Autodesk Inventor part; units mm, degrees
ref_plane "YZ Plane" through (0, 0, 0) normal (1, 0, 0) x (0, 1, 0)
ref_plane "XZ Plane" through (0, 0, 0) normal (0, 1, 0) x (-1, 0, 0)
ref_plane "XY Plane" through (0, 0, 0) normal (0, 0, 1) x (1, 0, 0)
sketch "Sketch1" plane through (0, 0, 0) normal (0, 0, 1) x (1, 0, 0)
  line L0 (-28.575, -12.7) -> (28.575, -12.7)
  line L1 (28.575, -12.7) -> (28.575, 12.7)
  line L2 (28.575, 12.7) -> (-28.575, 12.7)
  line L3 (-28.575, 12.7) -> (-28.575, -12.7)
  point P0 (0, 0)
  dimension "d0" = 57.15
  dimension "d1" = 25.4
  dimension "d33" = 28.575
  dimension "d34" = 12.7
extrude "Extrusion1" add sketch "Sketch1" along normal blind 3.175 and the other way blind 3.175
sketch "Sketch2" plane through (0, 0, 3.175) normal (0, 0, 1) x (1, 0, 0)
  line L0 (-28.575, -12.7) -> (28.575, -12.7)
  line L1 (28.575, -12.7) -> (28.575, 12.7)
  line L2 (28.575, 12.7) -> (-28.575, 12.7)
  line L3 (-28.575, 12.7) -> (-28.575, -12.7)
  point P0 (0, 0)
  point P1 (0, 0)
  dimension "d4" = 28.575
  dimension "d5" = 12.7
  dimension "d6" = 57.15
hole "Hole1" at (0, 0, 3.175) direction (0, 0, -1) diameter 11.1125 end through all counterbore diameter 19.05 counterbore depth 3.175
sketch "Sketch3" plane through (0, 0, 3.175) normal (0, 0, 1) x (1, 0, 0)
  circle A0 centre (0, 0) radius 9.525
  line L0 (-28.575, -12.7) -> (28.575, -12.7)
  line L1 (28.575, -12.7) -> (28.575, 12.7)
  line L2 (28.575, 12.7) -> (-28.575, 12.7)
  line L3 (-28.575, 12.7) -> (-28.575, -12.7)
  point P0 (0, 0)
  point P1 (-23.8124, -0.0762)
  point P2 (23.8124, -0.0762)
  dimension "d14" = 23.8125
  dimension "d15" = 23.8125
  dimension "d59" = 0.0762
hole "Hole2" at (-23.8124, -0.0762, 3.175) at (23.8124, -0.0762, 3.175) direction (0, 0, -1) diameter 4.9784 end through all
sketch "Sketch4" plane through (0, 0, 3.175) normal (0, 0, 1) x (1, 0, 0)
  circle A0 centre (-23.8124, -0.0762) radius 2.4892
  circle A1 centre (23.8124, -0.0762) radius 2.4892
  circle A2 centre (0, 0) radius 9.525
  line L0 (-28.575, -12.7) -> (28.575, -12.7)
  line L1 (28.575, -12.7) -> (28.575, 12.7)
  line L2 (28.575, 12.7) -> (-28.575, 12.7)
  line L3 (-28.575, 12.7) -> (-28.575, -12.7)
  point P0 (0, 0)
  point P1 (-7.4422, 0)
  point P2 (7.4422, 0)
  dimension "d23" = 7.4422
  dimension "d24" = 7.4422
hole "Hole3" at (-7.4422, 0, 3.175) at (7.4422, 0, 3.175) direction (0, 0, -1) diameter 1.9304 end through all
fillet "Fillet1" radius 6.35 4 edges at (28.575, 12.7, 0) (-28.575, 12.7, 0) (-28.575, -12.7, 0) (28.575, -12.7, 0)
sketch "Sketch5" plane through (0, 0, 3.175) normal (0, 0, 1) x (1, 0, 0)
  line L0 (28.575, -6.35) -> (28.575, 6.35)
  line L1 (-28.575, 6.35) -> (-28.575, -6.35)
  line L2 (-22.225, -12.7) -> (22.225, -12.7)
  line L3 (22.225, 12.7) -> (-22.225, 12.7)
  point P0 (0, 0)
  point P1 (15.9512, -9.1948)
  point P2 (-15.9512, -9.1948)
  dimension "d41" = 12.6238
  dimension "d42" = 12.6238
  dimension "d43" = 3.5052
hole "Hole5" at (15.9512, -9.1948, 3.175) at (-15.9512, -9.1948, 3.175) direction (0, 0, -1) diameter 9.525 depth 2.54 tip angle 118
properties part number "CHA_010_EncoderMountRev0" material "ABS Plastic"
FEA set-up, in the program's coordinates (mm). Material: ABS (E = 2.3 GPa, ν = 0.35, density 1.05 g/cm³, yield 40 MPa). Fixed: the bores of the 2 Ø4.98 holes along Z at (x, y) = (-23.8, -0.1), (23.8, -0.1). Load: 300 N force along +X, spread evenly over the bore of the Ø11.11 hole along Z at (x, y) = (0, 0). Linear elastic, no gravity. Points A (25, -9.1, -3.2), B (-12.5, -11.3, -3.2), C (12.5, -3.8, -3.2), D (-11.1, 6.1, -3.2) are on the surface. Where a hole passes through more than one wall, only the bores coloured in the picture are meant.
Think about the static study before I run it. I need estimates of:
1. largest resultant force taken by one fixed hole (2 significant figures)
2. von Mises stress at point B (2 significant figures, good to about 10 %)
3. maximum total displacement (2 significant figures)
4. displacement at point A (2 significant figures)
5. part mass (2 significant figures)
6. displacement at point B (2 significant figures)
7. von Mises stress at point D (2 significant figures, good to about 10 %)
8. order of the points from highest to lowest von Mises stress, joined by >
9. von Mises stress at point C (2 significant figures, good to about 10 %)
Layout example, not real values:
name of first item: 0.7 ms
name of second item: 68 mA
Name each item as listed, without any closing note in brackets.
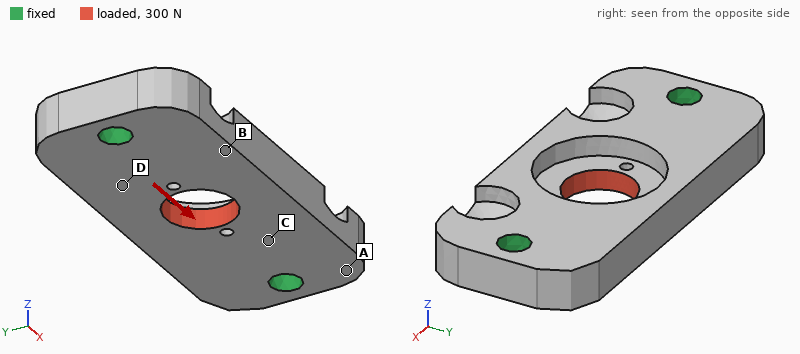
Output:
largest resultant force taken by one fixed hole: 150 N
von Mises stress at point B: 1.3 MPa
maximum total displacement: 24 µm
displacement at point A: 6.4 µm
part mass: 7.4 g
displacement at point B: 11 µm
von Mises stress at point D: 1.9 MPa
order of the points from highest to lowest von Mises stress, joined by >: C > D > B > A
von Mises stress at point C: 2.6 MPa
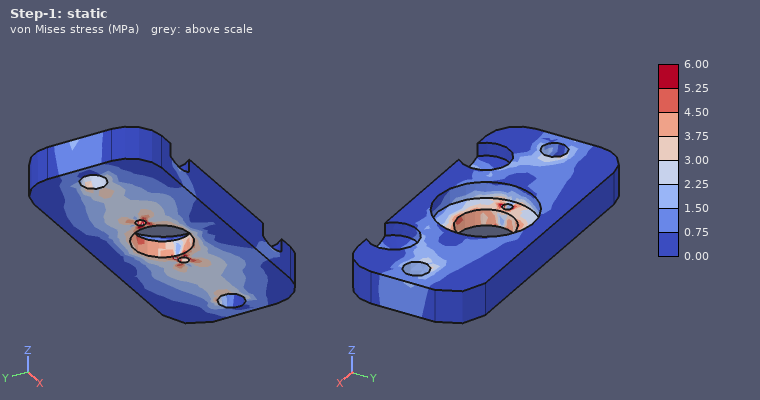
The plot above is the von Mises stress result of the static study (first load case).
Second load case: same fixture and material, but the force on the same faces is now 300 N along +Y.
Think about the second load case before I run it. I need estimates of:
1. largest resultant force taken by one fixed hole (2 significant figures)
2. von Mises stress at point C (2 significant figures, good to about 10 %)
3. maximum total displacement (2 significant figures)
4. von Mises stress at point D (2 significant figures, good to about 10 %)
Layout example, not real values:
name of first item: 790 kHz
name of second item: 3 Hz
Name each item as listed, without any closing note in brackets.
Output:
largest resultant force taken by one fixed hole: 150 N
von Mises stress at point C: 2.8 MPa
maximum total displacement: 75 µm
von Mises stress at point D: 3.1 MPa
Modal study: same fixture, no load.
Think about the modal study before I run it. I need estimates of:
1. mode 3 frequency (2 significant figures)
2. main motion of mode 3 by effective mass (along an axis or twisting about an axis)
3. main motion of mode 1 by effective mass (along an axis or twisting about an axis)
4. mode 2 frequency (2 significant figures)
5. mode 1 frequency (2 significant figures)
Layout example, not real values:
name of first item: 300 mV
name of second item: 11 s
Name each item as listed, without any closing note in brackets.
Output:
mode 3 frequency: 7000 Hz
main motion of mode 3 by effective mass: along Y
main motion of mode 1 by effective mass: along Z
mode 2 frequency: 4000 Hz
mode 1 frequency: 3700 Hz
